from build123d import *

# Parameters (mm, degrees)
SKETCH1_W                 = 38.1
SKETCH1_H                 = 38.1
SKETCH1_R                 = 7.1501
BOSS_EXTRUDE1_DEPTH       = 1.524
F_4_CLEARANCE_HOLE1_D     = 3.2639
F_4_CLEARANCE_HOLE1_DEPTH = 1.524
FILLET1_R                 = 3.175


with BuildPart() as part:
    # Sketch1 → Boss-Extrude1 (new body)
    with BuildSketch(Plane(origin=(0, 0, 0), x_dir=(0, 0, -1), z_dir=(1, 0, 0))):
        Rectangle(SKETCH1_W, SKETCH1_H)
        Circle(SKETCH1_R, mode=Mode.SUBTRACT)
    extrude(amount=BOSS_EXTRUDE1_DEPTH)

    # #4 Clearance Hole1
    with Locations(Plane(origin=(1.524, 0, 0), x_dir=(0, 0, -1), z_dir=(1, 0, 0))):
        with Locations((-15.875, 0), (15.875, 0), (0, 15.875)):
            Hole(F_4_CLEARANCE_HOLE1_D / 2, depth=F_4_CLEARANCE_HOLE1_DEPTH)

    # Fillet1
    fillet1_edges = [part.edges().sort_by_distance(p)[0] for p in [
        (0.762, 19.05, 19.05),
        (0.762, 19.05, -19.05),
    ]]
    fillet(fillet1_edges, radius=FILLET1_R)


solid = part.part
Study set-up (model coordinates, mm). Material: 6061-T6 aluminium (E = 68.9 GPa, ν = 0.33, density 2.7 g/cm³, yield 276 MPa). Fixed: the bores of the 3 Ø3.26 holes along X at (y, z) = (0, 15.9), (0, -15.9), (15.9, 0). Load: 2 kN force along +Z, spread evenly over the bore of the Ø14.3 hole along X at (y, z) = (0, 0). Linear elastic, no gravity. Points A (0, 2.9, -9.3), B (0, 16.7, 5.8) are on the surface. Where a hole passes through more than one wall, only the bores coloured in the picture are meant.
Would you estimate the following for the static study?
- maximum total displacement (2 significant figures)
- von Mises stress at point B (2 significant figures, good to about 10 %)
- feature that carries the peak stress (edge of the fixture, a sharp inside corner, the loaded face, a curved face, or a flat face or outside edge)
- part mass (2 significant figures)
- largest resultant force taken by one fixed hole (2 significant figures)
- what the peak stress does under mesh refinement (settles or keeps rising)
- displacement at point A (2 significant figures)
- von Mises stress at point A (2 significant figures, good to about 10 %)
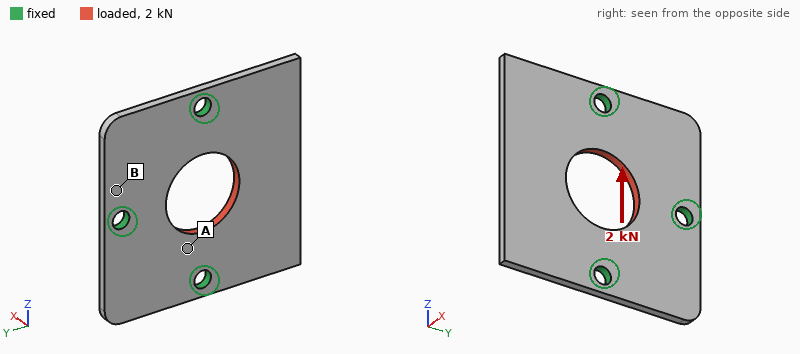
13 µm
15 MPa
edge of the fixture
5.2 g
810 N
keeps rising
4.2 µm
39 MPa
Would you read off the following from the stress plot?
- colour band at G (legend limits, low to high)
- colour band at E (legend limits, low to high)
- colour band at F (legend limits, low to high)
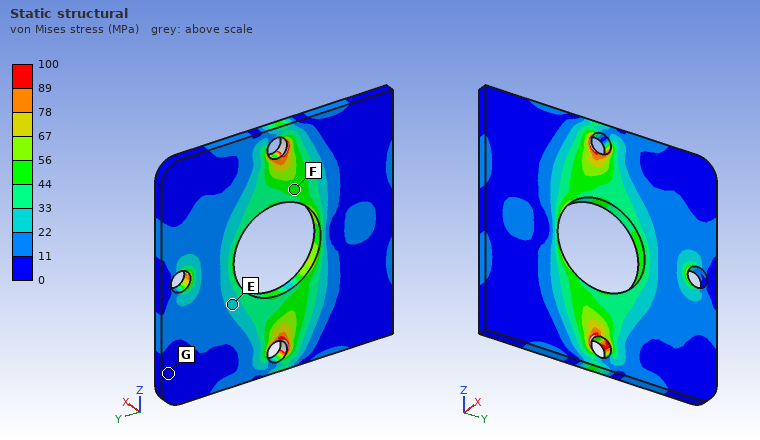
0 to 11 MPa
22 to 33 MPa
44 to 56 MPa
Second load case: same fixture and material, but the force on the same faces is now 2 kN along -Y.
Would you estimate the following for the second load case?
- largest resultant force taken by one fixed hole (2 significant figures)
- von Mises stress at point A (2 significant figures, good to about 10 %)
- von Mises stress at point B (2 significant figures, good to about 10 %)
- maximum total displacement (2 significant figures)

700 N
28 MPa
15 MPa
14 µm
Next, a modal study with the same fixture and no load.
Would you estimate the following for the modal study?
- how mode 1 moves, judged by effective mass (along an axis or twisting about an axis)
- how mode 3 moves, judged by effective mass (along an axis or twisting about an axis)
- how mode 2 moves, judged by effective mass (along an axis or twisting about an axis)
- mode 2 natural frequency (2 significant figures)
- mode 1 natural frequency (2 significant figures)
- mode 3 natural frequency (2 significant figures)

along X
along X
twisting about Y
5500 Hz
2800 Hz
7600 Hz
